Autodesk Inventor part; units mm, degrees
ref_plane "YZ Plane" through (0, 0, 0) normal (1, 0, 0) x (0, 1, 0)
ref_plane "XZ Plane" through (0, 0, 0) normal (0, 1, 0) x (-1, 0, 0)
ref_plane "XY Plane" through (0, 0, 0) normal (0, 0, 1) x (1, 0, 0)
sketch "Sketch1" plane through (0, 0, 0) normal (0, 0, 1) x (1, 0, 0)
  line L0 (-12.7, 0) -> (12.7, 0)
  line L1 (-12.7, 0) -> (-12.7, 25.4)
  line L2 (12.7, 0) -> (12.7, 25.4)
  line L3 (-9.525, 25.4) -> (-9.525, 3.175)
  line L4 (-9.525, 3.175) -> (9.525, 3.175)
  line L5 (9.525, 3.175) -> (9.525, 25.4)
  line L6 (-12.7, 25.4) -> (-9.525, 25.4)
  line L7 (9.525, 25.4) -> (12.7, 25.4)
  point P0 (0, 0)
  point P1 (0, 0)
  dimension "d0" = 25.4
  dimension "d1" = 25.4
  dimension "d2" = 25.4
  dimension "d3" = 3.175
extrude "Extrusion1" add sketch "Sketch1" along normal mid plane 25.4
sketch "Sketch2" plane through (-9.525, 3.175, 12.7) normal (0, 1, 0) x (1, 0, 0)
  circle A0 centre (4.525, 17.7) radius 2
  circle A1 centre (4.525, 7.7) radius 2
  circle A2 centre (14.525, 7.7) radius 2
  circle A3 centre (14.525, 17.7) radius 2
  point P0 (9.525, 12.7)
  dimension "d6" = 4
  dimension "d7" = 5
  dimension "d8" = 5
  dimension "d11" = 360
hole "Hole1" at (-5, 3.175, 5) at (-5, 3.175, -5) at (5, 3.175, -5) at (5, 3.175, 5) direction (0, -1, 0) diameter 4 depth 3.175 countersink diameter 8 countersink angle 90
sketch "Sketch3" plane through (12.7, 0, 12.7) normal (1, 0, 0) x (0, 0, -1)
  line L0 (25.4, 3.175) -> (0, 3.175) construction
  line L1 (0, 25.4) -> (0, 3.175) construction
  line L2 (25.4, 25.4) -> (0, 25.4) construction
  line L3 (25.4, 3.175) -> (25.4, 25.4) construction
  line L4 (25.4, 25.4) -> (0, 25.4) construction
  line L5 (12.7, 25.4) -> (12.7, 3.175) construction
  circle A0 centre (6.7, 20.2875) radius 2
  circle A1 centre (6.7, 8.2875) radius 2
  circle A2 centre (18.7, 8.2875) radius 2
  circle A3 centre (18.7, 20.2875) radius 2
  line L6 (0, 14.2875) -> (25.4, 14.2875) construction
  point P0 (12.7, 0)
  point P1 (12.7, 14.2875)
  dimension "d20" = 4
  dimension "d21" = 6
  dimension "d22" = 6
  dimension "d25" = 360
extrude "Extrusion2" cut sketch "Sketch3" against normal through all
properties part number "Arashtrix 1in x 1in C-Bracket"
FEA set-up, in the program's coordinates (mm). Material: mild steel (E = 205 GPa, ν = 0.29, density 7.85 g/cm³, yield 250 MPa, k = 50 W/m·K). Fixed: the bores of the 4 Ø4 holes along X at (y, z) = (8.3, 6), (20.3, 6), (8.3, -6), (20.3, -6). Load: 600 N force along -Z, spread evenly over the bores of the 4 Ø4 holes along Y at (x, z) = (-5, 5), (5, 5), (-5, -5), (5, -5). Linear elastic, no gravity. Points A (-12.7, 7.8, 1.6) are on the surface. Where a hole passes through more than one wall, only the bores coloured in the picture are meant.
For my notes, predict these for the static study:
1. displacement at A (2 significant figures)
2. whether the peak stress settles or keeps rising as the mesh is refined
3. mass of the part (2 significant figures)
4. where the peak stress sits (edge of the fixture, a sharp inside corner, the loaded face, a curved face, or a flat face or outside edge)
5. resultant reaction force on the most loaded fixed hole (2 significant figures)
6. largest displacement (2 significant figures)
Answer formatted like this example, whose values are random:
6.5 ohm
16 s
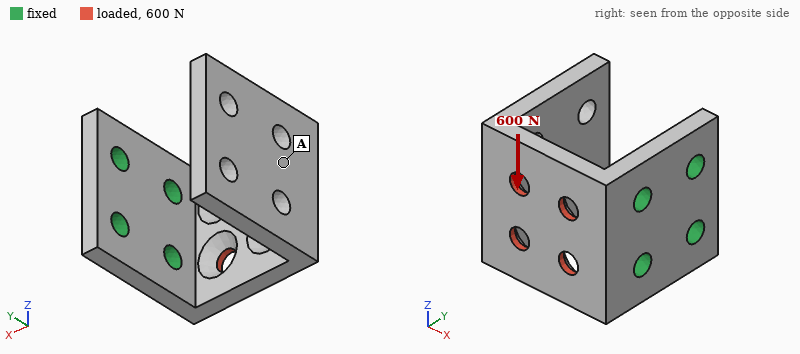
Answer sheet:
17 µm
keeps rising
39 g
edge of the fixture
570 N
23 µm
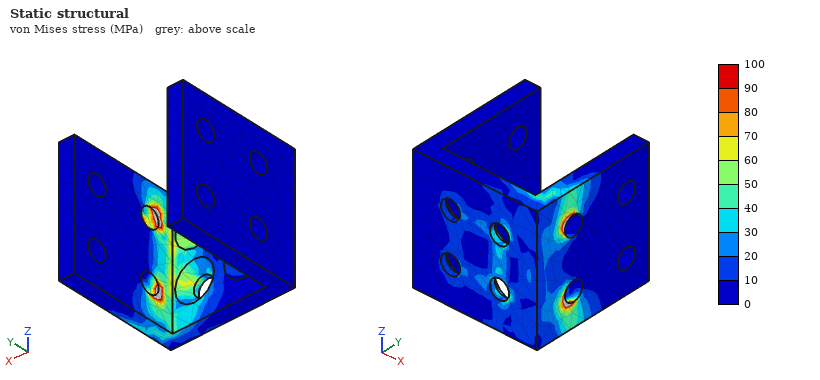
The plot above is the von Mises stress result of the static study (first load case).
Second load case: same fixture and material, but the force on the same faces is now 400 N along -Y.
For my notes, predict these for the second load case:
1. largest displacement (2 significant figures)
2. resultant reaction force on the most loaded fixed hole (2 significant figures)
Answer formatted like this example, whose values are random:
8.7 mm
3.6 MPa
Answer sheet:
0.13 mm
190 N
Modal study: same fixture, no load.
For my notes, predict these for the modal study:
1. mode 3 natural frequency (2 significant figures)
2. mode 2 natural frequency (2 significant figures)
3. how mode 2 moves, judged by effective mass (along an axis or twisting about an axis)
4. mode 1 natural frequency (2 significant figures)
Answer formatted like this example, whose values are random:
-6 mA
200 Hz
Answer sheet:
3700 Hz
2300 Hz
along Z
1300 Hz
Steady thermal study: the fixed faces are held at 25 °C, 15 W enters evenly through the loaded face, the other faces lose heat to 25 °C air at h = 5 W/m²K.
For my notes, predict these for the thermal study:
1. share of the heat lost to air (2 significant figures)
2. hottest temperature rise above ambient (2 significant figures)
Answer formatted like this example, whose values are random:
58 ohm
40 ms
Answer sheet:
5.6 %
75 K
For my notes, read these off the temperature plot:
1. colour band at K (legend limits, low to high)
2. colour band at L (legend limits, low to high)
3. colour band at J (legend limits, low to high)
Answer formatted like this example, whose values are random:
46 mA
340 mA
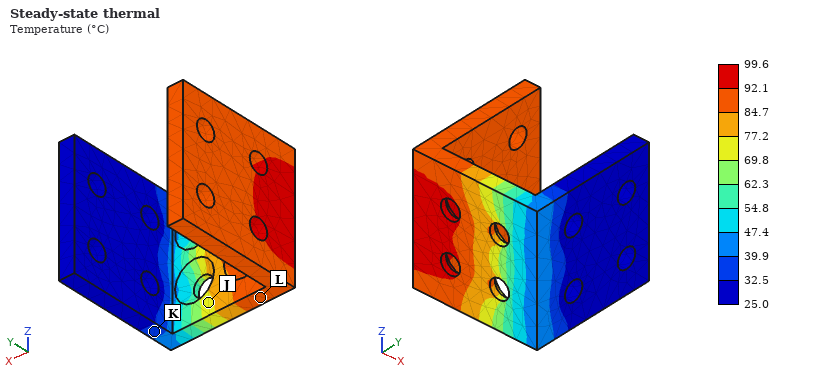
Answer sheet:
32.5 to 39.9 °C
84.7 to 92.1 °C
69.8 to 77.2 °C
